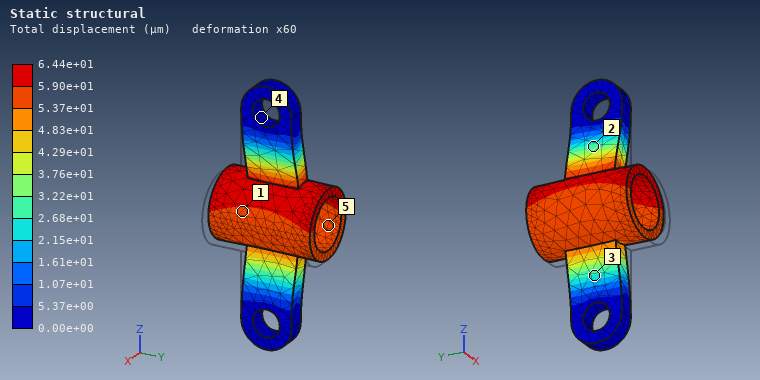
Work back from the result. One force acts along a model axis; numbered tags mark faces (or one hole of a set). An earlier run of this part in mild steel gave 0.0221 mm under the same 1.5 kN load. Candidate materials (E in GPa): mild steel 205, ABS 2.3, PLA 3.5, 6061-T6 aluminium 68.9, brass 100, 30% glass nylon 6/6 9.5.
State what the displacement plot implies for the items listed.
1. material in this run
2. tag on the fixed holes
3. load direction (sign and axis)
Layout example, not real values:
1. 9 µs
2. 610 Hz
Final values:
1. 6061-T6 aluminium
2. 4
3. -X
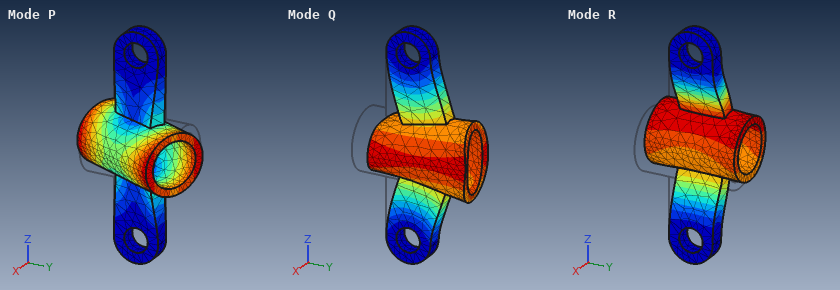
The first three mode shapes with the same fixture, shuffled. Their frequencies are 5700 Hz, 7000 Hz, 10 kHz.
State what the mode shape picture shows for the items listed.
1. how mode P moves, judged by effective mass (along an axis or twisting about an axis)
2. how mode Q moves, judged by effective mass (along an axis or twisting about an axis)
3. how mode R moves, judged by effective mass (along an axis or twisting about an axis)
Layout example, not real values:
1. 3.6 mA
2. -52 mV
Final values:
1. twisting about Z
2. along Y
3. along X
